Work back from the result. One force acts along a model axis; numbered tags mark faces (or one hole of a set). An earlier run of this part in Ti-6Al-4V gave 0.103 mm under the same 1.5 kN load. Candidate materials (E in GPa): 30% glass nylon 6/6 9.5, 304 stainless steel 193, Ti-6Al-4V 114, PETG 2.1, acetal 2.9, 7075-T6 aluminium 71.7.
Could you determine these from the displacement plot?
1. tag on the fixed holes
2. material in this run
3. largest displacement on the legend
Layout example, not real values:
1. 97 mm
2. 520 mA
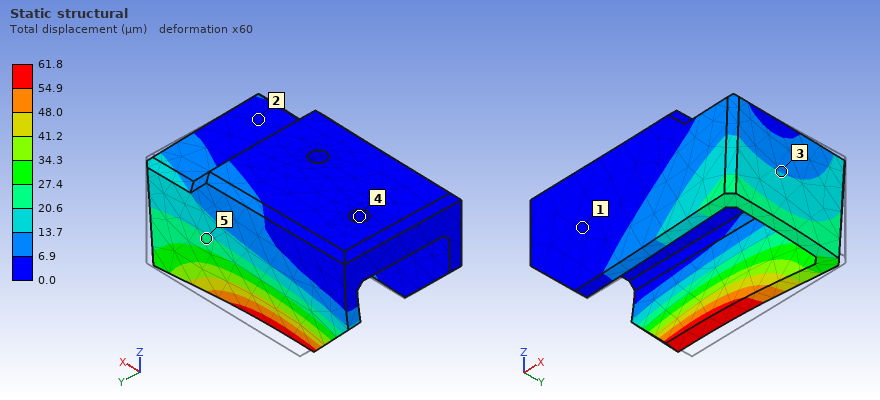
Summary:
1. 4
2. 304 stainless steel
3. 61.8 µm
